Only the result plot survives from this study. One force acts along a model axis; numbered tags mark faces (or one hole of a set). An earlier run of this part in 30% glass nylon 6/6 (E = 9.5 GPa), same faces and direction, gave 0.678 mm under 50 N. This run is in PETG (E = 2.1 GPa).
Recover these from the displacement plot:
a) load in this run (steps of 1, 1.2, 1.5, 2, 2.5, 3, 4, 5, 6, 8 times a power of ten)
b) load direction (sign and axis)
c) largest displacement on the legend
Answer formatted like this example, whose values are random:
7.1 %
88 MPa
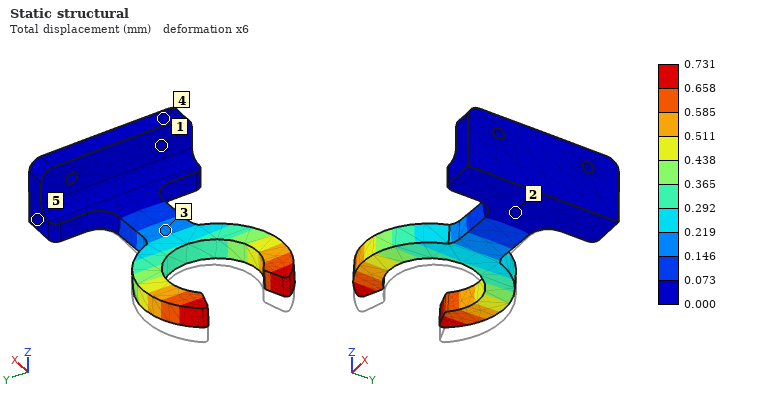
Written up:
12 N
+Z
0.731 mm
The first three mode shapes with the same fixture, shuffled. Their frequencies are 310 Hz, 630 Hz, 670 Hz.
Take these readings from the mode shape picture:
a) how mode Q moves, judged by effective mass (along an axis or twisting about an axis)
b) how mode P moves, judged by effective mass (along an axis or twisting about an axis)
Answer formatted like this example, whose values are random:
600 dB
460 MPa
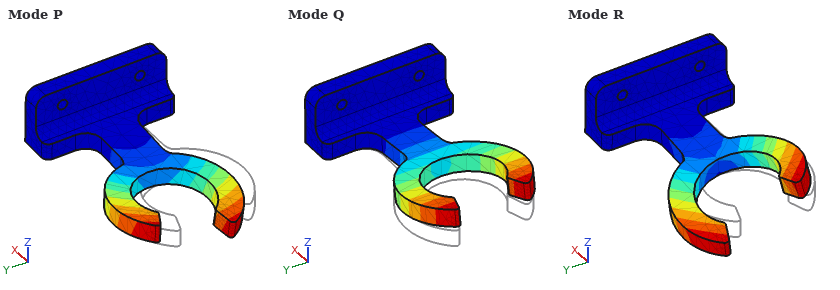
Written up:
along Z
along Y
